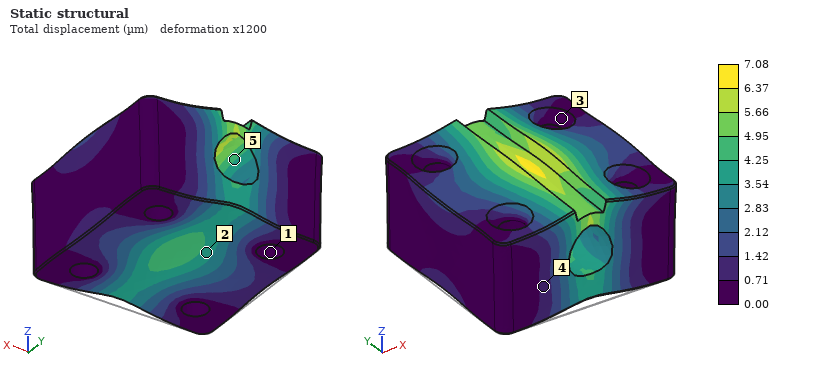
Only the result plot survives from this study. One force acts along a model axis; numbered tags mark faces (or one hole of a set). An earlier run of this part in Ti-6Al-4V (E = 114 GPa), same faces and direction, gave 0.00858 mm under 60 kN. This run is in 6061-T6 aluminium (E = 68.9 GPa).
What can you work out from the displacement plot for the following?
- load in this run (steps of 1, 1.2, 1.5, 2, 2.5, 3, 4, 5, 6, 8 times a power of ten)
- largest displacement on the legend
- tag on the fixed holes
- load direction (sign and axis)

30 kN
7.08 µm
1
+Z
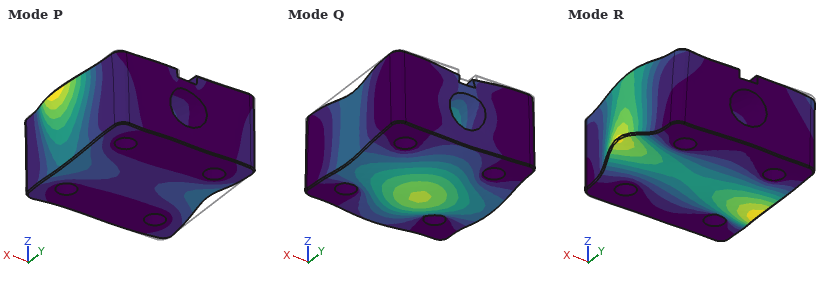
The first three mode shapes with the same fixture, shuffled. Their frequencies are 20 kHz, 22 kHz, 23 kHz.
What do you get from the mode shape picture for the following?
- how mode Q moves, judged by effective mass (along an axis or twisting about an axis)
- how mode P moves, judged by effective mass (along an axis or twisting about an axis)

along Z
along X
